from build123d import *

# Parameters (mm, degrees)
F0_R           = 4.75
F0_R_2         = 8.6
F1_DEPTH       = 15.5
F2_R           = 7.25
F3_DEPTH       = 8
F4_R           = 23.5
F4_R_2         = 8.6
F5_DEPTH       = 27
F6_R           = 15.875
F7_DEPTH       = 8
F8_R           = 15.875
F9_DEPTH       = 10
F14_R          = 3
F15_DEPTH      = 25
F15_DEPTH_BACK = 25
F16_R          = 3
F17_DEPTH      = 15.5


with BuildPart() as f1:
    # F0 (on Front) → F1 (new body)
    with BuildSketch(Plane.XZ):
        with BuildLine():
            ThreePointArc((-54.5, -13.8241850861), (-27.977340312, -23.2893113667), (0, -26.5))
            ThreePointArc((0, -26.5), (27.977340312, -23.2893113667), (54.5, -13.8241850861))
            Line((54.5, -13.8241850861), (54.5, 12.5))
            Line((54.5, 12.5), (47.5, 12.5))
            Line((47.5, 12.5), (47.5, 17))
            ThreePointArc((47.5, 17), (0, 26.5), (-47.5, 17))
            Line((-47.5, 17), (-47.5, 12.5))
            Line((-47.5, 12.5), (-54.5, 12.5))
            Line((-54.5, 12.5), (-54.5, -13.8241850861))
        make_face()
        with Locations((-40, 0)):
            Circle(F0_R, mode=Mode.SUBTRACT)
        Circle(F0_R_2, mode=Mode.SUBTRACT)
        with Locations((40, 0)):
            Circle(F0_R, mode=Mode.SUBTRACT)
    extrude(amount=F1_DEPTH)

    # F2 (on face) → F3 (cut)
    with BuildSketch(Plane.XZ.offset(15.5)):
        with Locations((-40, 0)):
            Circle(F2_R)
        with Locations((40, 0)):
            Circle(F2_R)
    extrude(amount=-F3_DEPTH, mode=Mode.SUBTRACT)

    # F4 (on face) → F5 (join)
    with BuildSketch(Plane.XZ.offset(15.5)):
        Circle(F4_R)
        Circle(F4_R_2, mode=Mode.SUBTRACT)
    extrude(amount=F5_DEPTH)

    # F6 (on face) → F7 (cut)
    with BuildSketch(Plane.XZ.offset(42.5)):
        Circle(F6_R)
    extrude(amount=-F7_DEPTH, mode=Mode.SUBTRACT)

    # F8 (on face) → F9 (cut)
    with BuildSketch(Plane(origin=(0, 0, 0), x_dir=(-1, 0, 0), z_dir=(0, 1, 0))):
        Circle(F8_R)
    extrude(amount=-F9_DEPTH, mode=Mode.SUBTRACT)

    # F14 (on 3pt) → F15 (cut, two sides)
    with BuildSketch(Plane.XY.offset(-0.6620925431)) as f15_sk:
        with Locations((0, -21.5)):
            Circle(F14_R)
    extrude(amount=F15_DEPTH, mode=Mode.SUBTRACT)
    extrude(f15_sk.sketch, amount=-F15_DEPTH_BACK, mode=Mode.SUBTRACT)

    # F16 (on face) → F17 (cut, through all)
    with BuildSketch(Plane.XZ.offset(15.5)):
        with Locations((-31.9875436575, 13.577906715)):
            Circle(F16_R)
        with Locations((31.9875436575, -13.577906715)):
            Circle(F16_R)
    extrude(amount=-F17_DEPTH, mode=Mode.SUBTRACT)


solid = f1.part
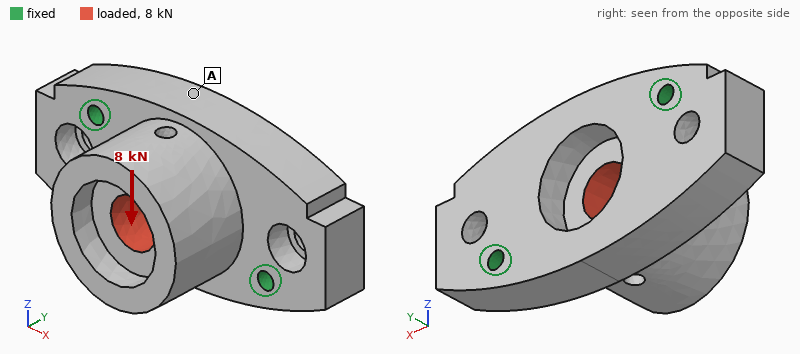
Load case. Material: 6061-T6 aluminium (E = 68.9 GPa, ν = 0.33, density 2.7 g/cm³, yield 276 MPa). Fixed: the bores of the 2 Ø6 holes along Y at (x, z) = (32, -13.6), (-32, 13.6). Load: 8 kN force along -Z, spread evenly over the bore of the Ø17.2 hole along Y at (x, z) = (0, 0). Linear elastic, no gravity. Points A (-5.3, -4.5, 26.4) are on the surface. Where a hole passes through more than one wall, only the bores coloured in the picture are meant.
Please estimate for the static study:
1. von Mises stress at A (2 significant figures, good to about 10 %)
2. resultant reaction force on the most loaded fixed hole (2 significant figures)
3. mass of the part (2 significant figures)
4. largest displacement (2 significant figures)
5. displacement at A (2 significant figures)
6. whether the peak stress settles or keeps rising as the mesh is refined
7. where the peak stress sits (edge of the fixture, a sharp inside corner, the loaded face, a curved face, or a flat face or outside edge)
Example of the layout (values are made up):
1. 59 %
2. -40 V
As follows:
1. 18 MPa
2. 4.1 kN
3. 260 g
4. 66 µm
5. 30 µm
6. keeps rising
7. edge of the fixture
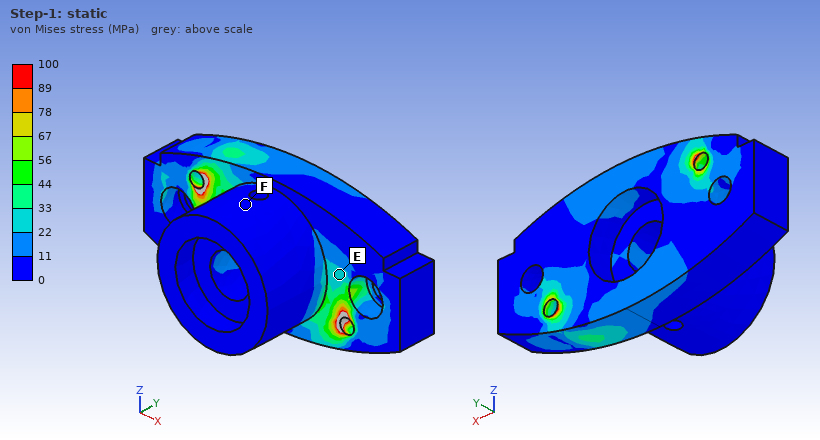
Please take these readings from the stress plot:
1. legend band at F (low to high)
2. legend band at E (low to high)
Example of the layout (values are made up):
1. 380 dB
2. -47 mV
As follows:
1. 0 to 11 MPa
2. 22 to 33 MPa
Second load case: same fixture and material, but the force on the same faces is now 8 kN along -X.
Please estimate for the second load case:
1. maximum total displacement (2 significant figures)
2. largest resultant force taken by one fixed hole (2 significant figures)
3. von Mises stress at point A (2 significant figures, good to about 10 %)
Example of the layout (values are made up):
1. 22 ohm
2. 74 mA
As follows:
1. 28 µm
2. 4.3 kN
3. 7.9 MPa
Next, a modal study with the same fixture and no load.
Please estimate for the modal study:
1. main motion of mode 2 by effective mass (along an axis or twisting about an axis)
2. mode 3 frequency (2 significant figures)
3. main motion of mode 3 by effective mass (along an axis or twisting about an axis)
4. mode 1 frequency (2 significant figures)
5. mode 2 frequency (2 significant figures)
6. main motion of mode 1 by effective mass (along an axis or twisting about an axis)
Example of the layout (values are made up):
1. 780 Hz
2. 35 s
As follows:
1. along Y
2. 11 kHz
3. along Z
4. 4400 Hz
5. 8300 Hz
6. along Z
